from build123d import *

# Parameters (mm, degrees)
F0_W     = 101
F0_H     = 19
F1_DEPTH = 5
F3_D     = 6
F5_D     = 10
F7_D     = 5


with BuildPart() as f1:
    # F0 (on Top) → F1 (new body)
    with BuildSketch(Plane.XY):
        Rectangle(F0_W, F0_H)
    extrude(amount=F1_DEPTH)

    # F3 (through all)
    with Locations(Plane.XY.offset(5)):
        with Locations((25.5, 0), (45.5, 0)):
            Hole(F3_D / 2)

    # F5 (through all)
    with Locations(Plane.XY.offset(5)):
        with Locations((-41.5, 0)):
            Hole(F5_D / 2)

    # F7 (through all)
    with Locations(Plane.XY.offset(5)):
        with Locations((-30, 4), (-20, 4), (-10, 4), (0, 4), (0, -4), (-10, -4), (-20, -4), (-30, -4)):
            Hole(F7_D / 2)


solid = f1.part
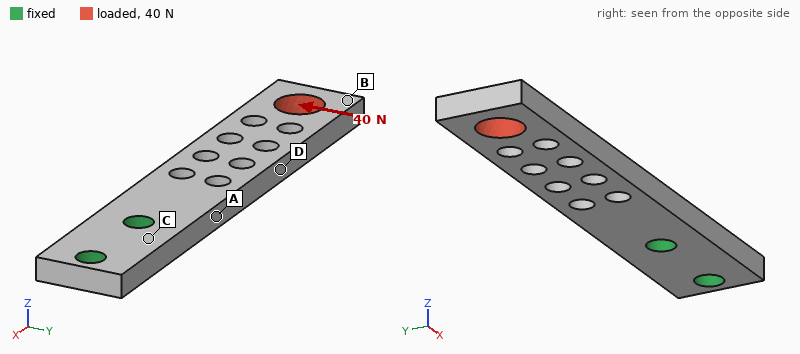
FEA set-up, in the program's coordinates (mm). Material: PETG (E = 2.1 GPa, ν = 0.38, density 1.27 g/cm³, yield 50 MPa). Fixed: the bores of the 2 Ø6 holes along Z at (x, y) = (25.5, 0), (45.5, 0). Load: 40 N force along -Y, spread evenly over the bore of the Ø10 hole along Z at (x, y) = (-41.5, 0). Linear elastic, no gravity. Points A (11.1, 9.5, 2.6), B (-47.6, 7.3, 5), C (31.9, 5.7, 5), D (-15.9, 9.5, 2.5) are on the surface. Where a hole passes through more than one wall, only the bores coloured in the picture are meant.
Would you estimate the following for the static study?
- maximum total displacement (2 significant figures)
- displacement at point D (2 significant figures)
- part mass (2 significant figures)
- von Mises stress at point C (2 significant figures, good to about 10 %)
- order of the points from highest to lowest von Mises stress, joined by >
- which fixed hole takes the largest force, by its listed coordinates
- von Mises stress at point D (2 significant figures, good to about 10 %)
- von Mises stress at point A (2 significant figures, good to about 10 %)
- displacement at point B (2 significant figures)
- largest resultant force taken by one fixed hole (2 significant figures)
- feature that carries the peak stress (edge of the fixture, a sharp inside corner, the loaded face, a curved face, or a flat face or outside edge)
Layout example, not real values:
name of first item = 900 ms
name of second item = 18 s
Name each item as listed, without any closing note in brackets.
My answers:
maximum total displacement = 1.2 mm
displacement at point D = 0.50 mm
part mass = 10 g
von Mises stress at point C = 2.4 MPa
order of the points from highest to lowest von Mises stress, joined by > = A > D > C > B
which fixed hole takes the largest force, by its listed coordinates = (25.5, 0)
von Mises stress at point D = 5.4 MPa
von Mises stress at point A = 7.2 MPa
displacement at point B = 1.1 mm
largest resultant force taken by one fixed hole = 110 N
feature that carries the peak stress = edge of the fixture
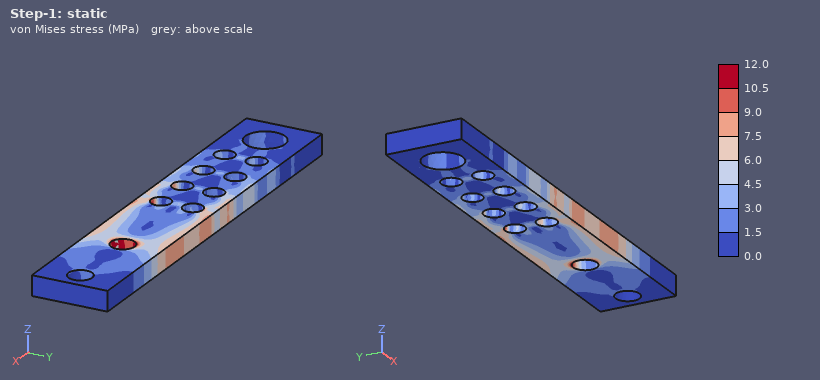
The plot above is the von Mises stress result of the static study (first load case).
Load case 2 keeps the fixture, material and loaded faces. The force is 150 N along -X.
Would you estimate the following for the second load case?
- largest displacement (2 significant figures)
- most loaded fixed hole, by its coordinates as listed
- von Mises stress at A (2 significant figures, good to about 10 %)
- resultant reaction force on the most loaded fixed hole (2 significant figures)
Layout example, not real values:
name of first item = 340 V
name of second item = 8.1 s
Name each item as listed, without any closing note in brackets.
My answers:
largest displacement = 91 µm
most loaded fixed hole, by its coordinates as listed = (25.5, 0)
von Mises stress at A = 1.7 MPa
resultant reaction force on the most loaded fixed hole = 130 N
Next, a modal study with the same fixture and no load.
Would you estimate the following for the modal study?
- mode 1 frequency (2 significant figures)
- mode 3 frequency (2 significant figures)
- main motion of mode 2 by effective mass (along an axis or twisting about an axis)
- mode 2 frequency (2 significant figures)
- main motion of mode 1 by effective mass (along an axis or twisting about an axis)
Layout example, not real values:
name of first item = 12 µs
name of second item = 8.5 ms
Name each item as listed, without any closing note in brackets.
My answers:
mode 1 frequency = 200 Hz
mode 3 frequency = 1100 Hz
main motion of mode 2 by effective mass = along Y
mode 2 frequency = 620 Hz
main motion of mode 1 by effective mass = along Z
